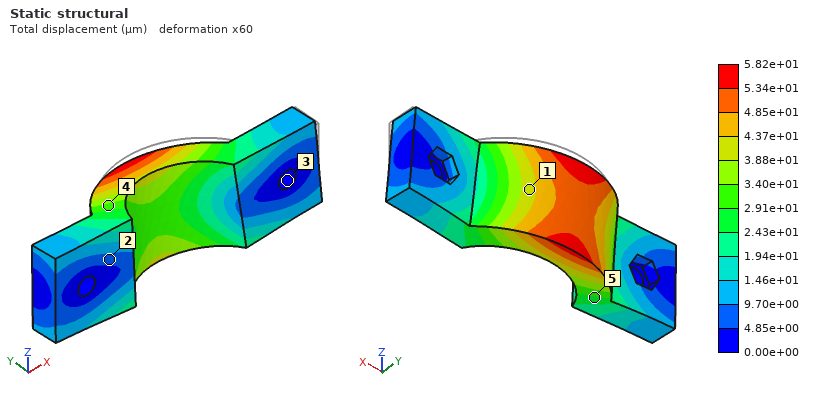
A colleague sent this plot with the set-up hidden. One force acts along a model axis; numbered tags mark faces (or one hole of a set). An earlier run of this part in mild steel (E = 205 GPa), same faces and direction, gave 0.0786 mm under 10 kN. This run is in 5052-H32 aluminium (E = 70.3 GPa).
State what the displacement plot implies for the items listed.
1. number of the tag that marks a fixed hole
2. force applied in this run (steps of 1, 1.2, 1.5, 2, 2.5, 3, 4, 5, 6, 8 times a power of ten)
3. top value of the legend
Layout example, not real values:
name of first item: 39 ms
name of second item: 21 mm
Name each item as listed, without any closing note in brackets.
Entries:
number of the tag that marks a fixed hole: 3
force applied in this run: 2.5 kN
top value of the legend: 5.82e+01 µm
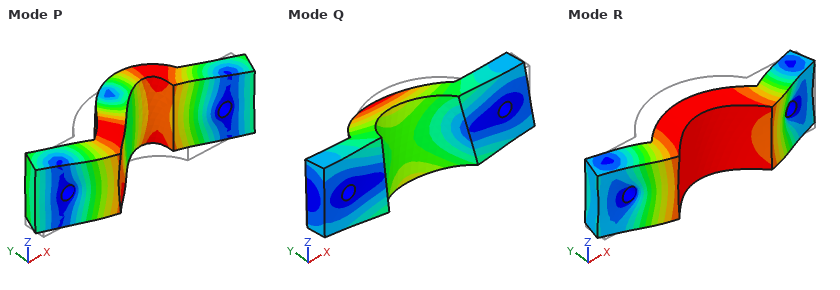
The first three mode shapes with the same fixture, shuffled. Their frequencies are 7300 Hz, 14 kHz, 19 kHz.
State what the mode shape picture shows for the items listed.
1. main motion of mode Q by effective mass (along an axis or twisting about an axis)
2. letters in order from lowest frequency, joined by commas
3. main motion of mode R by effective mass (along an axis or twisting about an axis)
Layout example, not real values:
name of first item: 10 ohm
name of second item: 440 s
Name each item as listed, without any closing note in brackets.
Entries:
main motion of mode Q by effective mass: along Z
letters in order from lowest frequency, joined by commas: Q, R, P
main motion of mode R by effective mass: along Y
